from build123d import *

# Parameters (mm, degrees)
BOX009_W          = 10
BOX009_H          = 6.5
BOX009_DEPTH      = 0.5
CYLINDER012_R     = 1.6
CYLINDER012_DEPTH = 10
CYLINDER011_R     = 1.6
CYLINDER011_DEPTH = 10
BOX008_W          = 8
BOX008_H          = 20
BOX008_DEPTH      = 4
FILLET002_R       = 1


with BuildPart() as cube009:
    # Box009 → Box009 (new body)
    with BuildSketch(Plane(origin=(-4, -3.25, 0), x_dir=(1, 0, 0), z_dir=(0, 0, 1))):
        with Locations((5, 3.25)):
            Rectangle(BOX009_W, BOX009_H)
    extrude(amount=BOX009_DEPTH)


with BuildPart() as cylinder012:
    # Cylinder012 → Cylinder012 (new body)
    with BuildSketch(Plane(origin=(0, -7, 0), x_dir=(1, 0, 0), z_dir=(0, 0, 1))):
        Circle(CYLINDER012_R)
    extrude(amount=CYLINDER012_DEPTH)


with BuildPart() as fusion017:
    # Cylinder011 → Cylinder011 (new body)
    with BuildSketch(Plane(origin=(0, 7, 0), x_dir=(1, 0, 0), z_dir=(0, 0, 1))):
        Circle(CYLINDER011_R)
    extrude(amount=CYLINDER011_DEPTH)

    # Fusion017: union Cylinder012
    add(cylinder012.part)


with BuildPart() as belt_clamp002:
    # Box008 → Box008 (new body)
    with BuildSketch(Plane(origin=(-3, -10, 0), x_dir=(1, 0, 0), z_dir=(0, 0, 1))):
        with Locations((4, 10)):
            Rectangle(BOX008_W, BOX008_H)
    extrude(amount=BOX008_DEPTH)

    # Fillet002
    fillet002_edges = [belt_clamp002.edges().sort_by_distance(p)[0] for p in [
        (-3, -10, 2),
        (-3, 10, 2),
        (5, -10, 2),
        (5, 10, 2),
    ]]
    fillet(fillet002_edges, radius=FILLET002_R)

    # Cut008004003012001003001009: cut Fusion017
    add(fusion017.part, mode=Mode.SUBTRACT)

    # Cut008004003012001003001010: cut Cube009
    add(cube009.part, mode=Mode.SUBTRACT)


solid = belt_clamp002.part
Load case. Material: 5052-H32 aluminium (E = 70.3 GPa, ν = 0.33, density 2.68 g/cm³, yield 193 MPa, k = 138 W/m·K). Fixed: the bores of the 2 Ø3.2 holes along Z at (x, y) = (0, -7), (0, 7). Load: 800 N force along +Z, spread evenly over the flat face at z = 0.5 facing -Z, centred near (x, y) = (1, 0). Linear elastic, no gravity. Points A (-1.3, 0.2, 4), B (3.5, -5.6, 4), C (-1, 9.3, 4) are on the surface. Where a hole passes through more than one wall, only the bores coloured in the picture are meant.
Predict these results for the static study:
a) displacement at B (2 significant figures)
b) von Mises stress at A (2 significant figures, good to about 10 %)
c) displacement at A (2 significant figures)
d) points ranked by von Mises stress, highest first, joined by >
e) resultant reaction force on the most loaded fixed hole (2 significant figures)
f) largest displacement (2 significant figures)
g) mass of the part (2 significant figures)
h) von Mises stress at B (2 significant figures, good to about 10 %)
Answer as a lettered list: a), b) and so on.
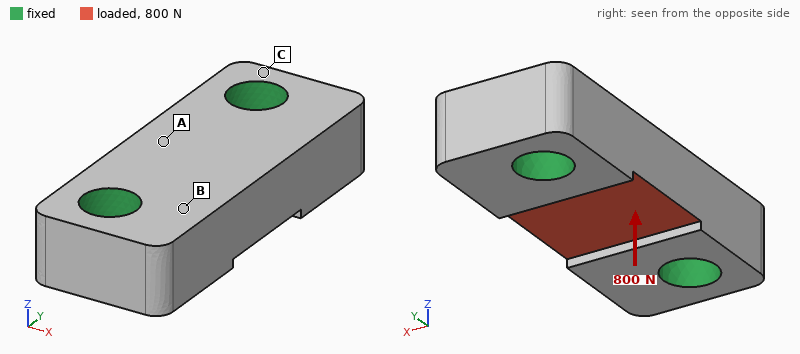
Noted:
a) 2.0 µm
b) 39 MPa
c) 4.4 µm
d) A > B > C
e) 400 N
f) 7.4 µm
g) 1.5 g
h) 19 MPa
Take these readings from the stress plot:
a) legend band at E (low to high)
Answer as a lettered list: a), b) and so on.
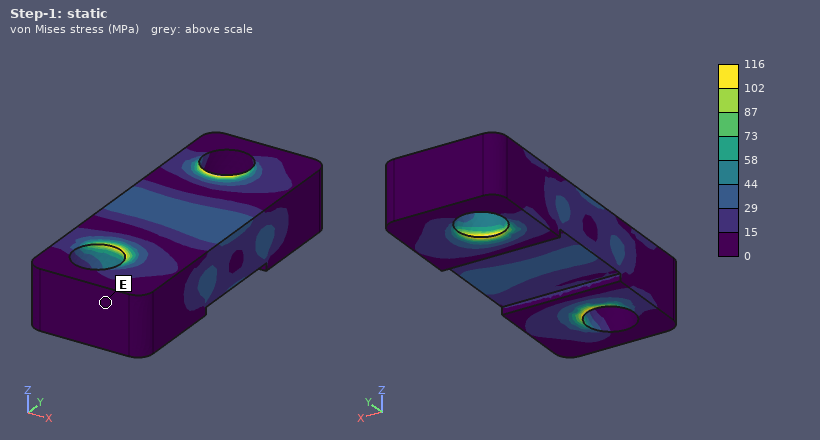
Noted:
a) 0 to 15 MPa
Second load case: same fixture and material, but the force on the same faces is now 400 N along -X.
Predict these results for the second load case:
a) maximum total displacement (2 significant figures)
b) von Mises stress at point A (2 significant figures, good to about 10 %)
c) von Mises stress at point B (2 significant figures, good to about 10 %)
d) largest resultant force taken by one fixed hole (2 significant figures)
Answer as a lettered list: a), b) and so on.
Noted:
a) 3.9 µm
b) 10 MPa
c) 4.9 MPa
d) 200 N
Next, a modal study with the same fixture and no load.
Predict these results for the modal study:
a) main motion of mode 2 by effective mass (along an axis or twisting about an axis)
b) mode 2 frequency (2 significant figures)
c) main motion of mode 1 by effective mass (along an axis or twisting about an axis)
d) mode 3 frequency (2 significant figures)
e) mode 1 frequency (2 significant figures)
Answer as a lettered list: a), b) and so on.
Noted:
a) along X
b) 100 kHz
c) along Z
d) 110 kHz
e) 80 kHz
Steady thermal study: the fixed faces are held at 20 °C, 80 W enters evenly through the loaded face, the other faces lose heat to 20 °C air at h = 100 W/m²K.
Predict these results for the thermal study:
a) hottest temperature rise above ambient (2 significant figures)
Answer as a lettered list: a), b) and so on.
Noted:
a) 59 K
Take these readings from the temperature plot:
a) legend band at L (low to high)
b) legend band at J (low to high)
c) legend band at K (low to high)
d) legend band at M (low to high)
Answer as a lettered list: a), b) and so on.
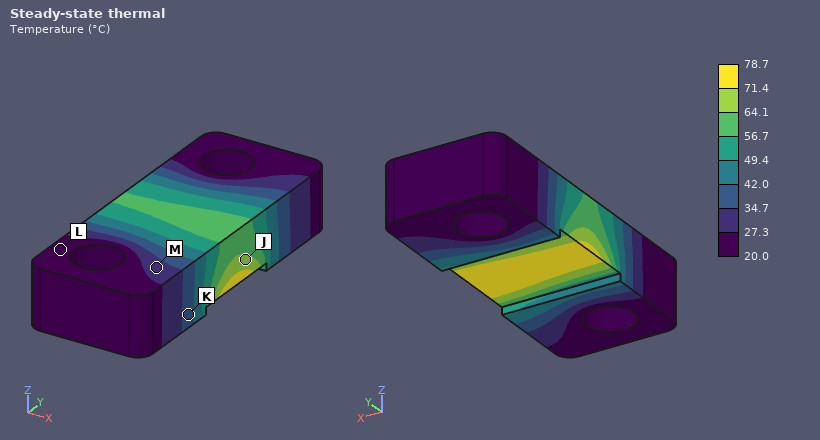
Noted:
a) 20.0 to 27.3 °C
b) 64.1 to 71.4 °C
c) 34.7 to 42.0 °C
d) 27.3 to 34.7 °C
